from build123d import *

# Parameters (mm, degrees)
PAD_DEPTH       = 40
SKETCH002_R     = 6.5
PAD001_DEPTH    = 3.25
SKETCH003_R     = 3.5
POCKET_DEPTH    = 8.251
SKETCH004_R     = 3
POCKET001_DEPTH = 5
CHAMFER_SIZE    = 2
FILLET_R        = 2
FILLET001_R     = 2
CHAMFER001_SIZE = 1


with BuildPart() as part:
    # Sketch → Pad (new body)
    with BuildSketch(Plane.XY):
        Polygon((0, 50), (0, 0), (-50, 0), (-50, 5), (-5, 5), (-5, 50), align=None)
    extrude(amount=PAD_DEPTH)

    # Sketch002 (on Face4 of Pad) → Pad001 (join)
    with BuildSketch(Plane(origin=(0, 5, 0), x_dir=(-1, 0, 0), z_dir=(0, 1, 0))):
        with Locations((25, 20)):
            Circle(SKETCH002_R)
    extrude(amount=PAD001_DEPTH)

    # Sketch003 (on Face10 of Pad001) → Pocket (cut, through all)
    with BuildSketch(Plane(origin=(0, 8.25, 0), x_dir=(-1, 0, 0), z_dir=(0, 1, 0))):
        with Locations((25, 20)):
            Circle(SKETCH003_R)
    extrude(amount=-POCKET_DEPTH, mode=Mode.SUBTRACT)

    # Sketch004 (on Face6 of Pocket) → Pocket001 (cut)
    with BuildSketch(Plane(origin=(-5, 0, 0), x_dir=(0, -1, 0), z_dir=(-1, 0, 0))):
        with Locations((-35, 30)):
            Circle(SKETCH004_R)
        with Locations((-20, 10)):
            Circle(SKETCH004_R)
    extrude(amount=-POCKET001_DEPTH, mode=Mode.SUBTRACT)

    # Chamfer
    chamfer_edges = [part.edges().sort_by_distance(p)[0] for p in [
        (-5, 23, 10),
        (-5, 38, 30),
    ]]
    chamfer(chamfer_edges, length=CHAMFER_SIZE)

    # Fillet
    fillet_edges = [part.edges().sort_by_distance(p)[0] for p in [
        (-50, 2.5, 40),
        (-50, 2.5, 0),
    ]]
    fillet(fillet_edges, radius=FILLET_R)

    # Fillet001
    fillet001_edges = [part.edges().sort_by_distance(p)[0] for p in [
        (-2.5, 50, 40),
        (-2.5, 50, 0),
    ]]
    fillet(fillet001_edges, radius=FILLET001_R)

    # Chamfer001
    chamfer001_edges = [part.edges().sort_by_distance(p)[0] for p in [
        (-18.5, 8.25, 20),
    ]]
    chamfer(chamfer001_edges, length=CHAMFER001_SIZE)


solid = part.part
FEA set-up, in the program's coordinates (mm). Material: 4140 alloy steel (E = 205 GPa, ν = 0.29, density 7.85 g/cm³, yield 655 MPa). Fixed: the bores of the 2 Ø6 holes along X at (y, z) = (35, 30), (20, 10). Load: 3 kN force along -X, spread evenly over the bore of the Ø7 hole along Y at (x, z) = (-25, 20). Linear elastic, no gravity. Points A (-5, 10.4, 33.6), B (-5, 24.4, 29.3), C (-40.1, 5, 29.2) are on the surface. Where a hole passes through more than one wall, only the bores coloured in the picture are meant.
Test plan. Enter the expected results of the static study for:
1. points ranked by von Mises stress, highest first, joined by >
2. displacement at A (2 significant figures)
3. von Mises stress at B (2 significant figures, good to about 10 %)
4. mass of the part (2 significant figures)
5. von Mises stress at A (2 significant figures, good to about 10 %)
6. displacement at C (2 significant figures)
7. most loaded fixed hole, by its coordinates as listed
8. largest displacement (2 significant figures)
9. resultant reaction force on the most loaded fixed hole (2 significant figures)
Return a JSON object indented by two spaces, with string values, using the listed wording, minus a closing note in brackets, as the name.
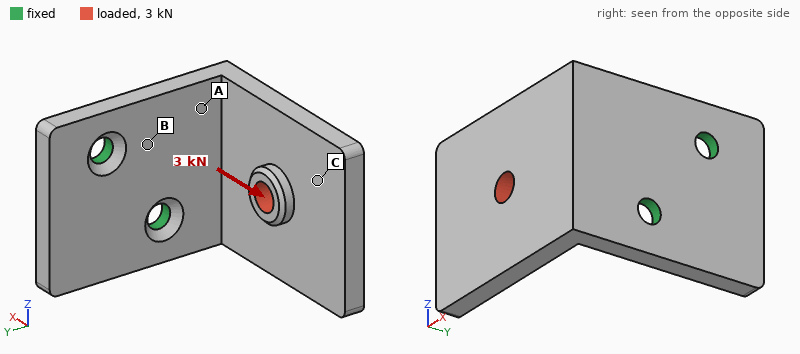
{
  "points ranked by von Mises stress, highest first, joined by >": "B > A > C",
  "displacement at A": "0.11 mm",
  "von Mises stress at B": "160 MPa",
  "mass of the part": "150 g",
  "von Mises stress at A": "76 MPa",
  "displacement at C": "0.31 mm",
  "most loaded fixed hole, by its coordinates as listed": "(20, 10)",
  "largest displacement": "0.40 mm",
  "resultant reaction force on the most loaded fixed hole": "2.9 kN"
}
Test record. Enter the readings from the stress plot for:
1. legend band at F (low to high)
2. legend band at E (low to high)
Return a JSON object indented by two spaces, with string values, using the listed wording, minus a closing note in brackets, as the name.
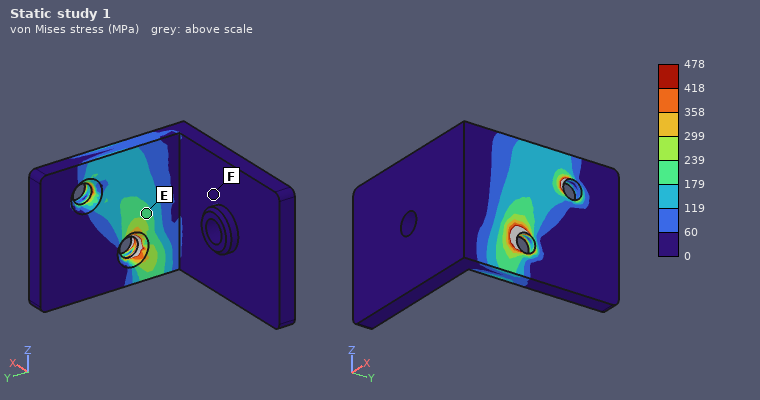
{
  "legend band at F": "0 to 60 MPa",
  "legend band at E": "179 to 239 MPa"
}
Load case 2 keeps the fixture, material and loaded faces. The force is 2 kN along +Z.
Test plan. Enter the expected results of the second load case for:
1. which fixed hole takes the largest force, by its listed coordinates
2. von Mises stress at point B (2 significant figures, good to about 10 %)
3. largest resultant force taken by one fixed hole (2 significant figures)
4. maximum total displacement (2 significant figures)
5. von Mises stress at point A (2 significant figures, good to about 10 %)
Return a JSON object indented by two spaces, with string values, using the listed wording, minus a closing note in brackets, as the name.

{
  "which fixed hole takes the largest force, by its listed coordinates": "(20, 10)",
  "von Mises stress at point B": "150 MPa",
  "largest resultant force taken by one fixed hole": "2.4 kN",
  "maximum total displacement": "0.34 mm",
  "von Mises stress at point A": "140 MPa"
}
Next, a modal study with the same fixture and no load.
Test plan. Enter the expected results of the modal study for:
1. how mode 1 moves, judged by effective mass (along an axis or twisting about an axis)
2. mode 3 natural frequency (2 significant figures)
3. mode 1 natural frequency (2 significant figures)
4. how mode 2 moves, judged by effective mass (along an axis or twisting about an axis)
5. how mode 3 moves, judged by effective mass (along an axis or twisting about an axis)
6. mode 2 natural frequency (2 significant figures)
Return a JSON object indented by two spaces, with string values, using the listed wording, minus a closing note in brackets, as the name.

{
  "how mode 1 moves, judged by effective mass": "along Y",
  "mode 3 natural frequency": "4000 Hz",
  "mode 1 natural frequency": "1100 Hz",
  "how mode 2 moves, judged by effective mass": "along Z",
  "how mode 3 moves, judged by effective mass": "along X",
  "mode 2 natural frequency": "1700 Hz"
}
